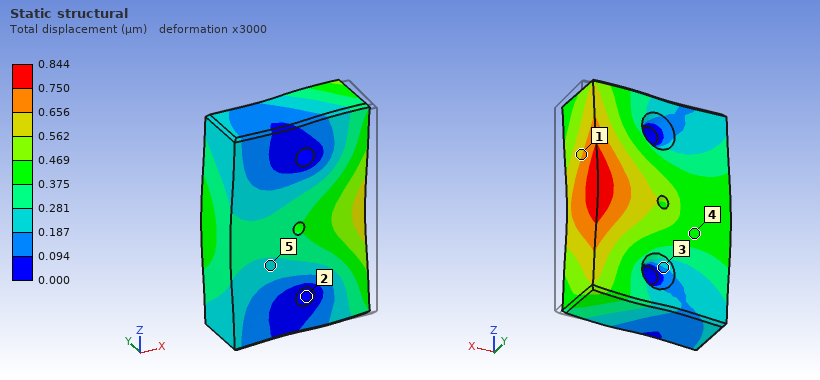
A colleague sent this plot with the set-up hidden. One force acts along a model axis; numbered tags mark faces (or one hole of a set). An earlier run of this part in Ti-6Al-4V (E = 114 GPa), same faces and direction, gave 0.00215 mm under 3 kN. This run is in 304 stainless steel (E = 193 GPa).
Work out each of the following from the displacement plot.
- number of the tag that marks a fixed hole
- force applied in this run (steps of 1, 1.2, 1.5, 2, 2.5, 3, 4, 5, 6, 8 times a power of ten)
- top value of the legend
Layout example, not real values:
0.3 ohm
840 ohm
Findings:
2
2 kN
0.844 µm
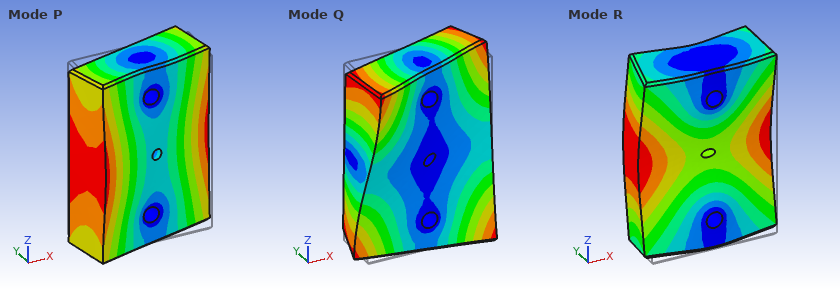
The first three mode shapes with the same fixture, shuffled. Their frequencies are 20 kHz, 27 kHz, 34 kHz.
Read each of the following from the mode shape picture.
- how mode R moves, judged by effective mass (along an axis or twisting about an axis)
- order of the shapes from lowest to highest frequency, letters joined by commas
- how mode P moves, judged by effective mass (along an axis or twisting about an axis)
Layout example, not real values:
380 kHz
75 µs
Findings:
along Y
P, R, Q
twisting about Z
